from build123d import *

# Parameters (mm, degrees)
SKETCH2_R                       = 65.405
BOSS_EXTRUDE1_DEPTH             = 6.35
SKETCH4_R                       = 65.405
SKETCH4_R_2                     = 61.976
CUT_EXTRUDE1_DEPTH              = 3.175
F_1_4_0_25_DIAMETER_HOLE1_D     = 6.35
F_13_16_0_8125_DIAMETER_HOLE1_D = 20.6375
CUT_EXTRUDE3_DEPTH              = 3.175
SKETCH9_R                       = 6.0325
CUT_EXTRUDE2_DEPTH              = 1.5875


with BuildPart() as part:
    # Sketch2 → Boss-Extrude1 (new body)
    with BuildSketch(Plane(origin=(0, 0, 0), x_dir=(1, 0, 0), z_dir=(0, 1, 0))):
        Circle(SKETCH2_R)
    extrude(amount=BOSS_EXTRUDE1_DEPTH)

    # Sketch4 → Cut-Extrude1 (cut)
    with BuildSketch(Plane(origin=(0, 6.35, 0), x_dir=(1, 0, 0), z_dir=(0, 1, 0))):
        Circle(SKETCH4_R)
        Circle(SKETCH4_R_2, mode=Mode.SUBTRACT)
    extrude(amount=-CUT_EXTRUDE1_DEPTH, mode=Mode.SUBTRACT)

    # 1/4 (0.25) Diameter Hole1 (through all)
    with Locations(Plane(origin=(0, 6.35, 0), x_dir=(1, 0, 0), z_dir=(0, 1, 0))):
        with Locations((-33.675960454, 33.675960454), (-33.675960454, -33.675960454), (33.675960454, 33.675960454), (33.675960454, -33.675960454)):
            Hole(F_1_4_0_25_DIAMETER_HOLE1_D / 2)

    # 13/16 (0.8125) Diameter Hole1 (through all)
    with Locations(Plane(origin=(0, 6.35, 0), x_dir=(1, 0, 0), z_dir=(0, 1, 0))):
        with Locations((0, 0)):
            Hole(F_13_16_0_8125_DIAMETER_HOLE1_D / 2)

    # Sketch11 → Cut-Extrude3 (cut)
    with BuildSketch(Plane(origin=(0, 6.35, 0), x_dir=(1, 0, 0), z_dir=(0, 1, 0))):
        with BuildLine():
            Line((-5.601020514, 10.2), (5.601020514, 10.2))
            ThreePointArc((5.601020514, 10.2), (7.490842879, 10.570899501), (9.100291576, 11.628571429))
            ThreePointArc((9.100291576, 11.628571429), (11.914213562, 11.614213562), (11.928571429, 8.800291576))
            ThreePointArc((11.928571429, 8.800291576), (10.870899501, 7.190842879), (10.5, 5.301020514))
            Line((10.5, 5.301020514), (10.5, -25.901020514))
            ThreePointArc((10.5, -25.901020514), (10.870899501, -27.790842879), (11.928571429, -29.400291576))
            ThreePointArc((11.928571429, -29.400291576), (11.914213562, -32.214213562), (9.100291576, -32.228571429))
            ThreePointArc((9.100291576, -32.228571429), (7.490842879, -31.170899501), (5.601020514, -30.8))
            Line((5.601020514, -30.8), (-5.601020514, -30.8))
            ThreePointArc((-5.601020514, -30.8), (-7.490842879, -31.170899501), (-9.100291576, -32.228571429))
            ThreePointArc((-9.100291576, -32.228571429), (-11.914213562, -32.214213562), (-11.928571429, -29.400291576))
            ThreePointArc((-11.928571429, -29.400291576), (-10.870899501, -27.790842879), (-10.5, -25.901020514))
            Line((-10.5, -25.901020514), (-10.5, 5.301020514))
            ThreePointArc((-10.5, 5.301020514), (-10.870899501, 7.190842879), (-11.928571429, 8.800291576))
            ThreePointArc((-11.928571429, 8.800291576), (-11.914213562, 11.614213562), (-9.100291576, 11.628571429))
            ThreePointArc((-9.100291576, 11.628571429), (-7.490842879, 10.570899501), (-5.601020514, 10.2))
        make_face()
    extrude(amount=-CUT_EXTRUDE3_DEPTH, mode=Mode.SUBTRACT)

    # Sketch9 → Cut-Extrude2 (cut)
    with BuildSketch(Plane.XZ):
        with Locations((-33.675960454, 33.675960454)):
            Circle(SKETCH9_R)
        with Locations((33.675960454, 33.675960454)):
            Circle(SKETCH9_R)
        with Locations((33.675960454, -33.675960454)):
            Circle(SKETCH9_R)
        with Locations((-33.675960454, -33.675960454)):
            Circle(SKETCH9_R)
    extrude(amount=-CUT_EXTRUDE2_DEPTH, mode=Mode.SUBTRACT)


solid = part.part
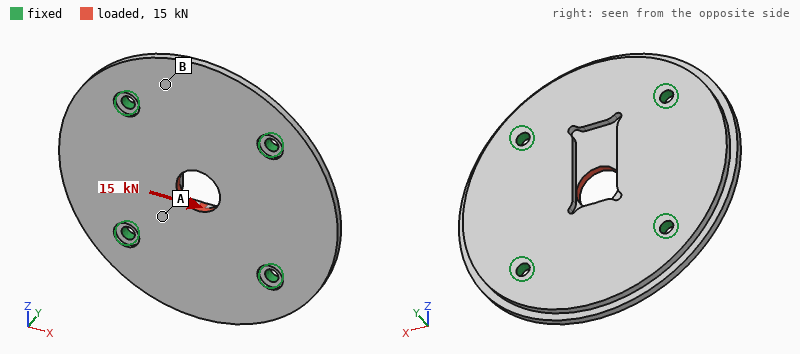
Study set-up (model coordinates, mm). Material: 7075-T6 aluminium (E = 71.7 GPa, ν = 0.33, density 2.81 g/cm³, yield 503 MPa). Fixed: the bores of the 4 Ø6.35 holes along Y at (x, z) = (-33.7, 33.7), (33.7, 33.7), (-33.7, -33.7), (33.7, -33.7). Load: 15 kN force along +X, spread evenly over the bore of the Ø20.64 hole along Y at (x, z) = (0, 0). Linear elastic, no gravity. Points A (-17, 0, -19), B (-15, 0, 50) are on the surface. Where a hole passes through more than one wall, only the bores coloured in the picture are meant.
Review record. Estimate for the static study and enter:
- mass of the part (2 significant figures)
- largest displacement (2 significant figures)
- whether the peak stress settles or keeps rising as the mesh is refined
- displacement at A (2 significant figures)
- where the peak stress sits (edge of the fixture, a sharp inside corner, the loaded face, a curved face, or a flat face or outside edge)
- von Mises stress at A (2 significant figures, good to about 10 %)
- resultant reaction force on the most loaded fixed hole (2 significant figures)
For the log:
210 g
32 µm
keeps rising
11 µm
a sharp inside corner
33 MPa
4.2 kN
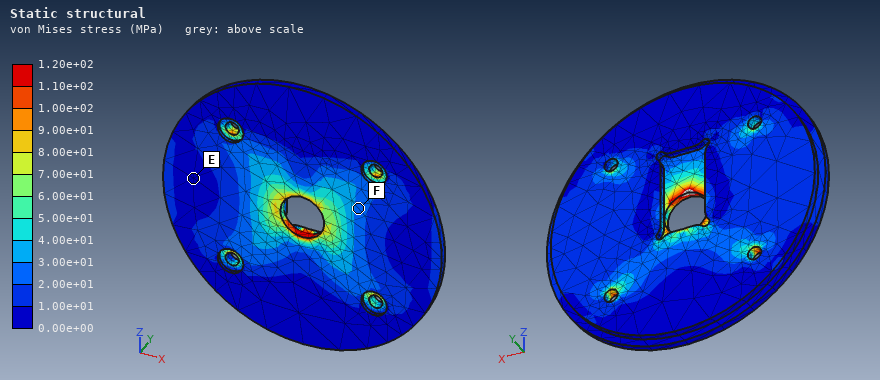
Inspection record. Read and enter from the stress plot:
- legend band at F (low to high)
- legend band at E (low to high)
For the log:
2.00e+01 to 3.00e+01 MPa
0.00e+00 to 1.00e+01 MPa
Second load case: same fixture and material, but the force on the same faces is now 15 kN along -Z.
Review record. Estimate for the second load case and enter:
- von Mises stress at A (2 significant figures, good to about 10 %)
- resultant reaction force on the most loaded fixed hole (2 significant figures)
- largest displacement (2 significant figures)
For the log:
31 MPa
4.0 kN
27 µm
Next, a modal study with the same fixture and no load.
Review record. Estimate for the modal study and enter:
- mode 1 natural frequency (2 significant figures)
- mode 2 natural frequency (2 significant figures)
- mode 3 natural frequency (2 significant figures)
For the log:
3700 Hz
4200 Hz
4200 Hz
